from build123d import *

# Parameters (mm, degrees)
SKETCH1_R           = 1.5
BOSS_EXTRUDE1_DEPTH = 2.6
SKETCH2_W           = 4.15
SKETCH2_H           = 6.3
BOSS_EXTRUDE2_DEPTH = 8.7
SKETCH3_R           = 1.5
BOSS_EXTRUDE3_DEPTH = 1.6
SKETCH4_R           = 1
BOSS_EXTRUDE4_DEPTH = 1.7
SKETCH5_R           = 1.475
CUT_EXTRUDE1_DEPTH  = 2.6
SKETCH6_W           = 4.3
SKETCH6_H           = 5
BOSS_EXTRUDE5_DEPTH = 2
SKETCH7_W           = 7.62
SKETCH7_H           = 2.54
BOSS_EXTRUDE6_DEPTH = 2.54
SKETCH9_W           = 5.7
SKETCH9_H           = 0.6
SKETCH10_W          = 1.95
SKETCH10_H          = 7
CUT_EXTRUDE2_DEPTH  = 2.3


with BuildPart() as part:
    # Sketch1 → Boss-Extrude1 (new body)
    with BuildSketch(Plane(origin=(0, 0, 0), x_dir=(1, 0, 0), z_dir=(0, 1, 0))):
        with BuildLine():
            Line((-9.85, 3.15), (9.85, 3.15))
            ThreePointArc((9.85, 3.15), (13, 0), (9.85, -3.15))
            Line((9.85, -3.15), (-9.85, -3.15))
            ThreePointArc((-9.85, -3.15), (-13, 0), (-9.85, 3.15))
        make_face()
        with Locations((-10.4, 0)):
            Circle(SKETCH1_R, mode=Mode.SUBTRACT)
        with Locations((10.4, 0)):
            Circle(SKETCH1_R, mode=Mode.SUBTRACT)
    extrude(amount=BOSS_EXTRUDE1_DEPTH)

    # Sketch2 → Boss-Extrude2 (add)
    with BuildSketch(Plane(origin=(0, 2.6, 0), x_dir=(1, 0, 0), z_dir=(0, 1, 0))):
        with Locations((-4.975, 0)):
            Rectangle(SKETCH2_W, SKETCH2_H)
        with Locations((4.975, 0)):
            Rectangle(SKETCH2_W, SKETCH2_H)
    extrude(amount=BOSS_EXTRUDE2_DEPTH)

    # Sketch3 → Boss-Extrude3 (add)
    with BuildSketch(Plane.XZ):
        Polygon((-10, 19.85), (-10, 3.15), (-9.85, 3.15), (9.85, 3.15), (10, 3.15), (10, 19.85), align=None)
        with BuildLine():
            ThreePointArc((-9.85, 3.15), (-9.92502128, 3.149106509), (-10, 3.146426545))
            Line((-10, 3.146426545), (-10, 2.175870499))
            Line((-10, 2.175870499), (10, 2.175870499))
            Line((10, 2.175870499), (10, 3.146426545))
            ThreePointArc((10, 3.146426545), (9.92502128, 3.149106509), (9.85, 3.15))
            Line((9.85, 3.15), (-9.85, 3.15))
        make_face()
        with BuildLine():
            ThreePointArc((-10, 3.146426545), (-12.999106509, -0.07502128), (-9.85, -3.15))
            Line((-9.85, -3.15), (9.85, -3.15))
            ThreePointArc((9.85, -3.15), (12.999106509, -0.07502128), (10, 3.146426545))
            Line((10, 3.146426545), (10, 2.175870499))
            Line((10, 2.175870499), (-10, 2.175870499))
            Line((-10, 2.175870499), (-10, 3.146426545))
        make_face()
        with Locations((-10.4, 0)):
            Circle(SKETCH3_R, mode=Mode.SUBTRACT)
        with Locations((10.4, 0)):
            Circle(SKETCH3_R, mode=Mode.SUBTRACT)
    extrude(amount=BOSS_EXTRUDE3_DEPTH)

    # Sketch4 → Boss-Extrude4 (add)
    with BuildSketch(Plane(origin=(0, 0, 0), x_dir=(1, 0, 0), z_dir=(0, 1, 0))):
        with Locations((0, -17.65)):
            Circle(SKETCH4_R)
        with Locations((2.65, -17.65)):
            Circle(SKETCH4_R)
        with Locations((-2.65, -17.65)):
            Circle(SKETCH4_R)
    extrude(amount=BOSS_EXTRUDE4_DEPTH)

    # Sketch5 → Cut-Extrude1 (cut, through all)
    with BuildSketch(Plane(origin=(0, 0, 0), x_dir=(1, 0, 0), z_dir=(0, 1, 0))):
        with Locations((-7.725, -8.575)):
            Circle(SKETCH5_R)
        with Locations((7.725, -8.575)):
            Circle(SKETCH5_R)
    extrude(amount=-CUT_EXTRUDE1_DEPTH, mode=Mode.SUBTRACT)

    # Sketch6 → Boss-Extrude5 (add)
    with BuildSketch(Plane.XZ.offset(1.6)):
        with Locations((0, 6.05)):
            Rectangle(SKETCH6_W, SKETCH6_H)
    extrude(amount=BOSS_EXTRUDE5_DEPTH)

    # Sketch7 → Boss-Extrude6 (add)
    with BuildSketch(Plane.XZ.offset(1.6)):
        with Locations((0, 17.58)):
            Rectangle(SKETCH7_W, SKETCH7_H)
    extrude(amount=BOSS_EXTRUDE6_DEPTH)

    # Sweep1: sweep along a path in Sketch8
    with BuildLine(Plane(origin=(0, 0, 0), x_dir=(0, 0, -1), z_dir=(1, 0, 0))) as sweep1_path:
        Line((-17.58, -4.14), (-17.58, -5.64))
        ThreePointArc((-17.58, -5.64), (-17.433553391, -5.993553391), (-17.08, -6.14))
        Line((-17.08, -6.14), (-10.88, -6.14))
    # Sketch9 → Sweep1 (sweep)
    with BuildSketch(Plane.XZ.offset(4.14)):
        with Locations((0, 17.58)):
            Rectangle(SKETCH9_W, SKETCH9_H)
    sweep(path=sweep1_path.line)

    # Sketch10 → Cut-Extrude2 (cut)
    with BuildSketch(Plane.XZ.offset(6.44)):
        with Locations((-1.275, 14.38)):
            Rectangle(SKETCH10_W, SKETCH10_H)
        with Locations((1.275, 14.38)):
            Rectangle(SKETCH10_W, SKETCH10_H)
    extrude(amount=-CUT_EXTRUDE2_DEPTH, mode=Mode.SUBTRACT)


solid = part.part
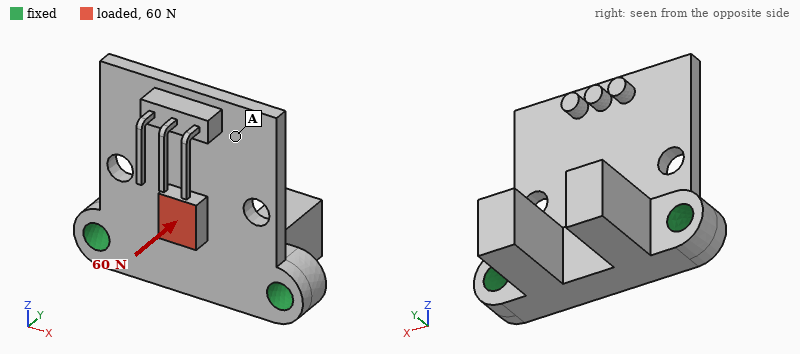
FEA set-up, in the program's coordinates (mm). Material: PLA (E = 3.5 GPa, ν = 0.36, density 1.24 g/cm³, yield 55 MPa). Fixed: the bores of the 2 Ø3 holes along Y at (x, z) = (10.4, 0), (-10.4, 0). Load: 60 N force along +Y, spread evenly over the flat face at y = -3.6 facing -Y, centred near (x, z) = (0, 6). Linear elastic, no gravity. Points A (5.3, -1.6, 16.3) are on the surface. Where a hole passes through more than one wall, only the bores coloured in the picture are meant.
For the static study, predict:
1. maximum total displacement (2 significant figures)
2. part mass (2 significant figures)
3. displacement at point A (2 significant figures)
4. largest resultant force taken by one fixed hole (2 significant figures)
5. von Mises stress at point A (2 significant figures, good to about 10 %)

0.43 mm
2.1 g
0.33 mm
30 N
2.1 MPa
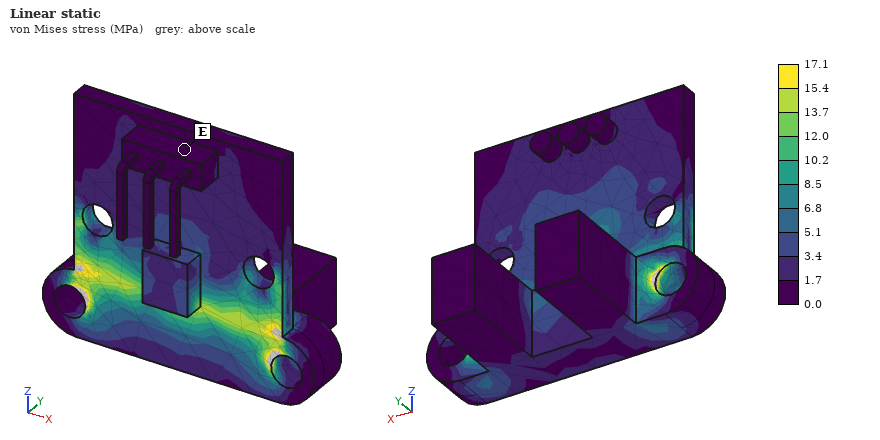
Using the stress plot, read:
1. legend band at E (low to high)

0.0 to 1.7 MPa
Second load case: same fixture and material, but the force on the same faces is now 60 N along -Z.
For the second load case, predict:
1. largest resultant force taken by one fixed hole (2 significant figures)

33 N
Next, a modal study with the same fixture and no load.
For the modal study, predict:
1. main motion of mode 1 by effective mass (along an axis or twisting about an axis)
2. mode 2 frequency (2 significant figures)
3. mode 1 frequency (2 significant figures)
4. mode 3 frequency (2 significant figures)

along Y
2100 Hz
1200 Hz
2200 Hz
